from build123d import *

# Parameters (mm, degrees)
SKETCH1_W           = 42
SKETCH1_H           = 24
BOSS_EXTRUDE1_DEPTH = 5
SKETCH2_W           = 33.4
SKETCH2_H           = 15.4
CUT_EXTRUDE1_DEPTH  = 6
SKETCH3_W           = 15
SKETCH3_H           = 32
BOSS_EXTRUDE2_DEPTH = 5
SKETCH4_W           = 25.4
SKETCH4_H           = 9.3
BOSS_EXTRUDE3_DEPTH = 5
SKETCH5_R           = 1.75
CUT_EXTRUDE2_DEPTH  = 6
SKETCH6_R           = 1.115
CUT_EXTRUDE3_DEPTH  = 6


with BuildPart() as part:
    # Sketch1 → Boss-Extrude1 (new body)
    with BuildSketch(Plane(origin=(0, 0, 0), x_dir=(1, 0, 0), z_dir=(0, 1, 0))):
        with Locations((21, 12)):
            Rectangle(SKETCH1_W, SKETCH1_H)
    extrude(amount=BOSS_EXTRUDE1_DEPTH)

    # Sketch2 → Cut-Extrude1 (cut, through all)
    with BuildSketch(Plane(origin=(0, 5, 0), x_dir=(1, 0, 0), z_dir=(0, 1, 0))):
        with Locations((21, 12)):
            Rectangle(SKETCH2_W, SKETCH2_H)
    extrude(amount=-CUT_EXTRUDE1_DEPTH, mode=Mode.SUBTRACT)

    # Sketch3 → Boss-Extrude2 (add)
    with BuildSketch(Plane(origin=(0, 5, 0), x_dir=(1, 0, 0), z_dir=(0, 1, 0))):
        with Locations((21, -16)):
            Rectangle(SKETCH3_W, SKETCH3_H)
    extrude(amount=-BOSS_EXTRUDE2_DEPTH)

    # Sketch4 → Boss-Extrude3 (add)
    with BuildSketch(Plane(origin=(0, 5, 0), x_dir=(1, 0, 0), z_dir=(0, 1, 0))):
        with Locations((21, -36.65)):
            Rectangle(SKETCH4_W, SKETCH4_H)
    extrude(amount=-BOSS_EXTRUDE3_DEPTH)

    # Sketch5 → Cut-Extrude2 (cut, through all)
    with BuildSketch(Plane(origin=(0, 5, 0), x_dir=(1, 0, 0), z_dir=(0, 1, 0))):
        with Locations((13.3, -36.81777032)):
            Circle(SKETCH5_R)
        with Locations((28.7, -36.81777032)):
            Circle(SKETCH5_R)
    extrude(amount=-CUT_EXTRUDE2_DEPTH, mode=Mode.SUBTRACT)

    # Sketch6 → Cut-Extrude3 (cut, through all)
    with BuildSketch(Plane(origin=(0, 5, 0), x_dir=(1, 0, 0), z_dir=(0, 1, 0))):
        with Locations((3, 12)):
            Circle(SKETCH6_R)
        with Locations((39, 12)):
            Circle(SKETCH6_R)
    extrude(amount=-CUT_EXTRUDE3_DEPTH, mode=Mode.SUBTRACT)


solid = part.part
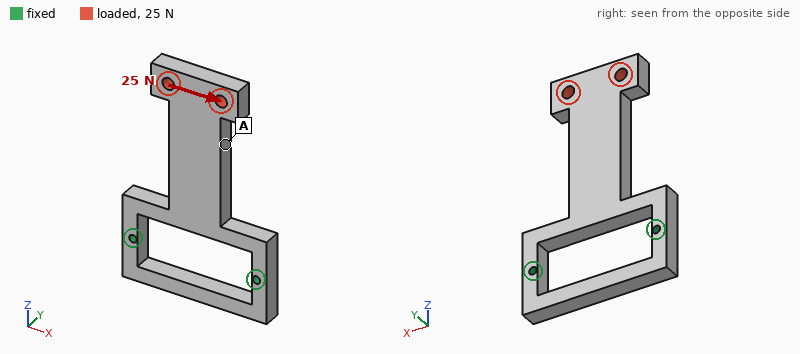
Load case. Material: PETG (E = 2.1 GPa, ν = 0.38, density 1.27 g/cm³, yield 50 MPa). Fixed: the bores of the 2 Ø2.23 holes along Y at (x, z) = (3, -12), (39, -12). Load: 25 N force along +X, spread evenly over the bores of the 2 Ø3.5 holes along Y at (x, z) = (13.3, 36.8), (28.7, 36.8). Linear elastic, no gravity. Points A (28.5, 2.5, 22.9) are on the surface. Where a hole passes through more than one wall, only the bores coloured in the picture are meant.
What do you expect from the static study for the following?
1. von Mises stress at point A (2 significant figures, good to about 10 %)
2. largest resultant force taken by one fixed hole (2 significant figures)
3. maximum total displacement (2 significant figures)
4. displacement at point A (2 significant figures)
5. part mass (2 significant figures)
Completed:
1.9 MPa
35 N
0.73 mm
0.38 mm
7.5 g
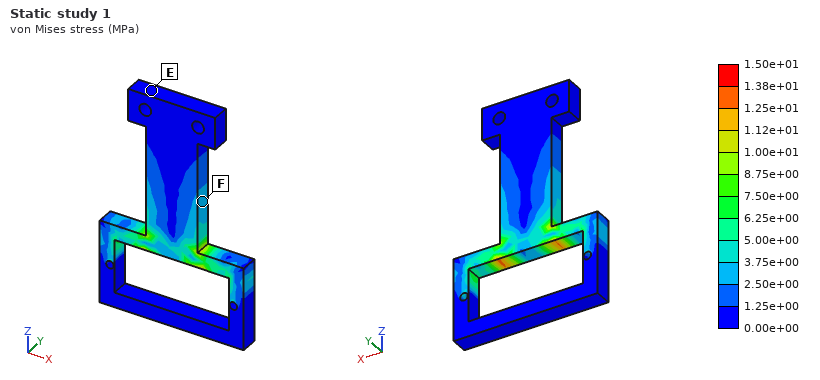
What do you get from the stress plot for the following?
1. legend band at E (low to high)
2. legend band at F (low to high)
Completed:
0.00e+00 to 1.25e+00 MPa
2.50e+00 to 3.75e+00 MPa
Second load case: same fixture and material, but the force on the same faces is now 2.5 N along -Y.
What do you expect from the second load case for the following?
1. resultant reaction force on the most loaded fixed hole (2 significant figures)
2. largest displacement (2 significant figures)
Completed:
1.3 N
0.90 mm
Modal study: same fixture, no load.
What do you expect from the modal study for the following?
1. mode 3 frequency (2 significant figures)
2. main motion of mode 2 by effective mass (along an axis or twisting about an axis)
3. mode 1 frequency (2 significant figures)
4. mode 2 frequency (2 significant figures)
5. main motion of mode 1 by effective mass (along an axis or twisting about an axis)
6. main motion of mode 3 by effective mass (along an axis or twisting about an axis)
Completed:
1500 Hz
along X
190 Hz
690 Hz
along Y
along Y
